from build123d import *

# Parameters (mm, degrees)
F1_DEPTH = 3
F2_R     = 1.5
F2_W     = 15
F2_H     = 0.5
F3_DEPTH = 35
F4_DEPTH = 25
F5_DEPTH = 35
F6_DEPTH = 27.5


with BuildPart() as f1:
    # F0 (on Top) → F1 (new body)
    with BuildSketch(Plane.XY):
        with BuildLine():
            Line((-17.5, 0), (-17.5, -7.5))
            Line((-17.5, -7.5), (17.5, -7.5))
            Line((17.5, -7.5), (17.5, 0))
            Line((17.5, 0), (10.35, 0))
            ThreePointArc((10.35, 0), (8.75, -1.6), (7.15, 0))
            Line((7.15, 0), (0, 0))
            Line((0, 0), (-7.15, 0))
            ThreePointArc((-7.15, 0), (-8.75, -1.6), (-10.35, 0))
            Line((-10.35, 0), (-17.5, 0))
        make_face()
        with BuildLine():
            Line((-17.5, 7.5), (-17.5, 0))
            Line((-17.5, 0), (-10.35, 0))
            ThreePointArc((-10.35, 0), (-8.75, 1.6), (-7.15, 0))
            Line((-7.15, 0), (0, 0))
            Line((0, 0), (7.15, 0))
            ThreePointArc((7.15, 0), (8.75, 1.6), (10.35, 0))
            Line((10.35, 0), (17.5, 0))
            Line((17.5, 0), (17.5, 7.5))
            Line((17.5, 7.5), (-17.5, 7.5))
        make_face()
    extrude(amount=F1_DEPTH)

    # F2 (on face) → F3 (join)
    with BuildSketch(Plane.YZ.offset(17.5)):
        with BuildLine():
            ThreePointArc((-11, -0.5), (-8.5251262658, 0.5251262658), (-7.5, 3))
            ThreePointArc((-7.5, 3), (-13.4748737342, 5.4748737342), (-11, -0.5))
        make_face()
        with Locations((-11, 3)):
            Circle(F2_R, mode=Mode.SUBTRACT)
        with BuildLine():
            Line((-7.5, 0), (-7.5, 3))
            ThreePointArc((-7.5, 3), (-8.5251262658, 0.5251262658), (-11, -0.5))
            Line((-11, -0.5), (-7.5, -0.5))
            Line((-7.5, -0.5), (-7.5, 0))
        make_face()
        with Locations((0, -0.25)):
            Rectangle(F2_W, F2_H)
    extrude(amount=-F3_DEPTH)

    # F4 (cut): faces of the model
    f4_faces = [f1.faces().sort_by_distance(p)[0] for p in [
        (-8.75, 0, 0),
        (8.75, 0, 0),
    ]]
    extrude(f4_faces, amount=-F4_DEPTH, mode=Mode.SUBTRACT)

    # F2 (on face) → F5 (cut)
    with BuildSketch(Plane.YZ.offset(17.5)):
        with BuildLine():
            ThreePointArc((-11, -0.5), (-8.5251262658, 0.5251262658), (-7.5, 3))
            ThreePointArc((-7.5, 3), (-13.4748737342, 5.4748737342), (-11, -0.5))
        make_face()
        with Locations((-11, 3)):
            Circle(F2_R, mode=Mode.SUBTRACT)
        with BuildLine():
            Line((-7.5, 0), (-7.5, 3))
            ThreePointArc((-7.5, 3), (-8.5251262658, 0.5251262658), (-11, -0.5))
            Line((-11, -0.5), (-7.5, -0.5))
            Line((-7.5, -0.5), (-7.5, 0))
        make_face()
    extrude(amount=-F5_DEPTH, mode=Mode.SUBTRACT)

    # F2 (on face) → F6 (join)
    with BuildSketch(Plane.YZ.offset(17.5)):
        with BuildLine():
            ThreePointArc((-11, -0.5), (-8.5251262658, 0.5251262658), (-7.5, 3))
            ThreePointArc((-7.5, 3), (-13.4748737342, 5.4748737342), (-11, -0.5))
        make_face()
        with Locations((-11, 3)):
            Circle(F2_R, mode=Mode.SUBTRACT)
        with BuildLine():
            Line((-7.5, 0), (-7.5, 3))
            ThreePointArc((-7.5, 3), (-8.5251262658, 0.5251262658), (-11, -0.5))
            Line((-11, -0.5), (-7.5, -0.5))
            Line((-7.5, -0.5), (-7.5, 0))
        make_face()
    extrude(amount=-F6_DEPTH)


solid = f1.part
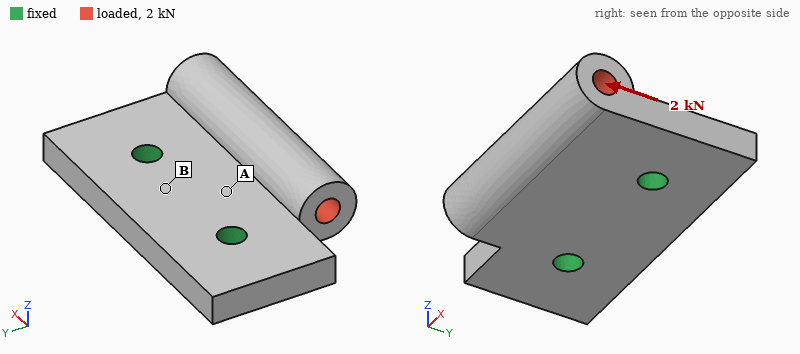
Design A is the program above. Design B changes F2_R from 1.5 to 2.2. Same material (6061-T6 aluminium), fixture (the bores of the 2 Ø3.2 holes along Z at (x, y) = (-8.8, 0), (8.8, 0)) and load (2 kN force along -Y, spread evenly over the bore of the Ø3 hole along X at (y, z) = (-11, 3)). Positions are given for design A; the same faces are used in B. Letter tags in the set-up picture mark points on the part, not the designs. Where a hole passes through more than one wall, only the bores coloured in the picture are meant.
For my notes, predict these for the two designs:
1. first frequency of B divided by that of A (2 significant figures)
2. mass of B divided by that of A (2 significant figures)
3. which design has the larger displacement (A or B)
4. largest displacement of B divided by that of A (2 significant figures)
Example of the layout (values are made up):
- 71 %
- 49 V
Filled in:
- 1.1
- 0.92
- B
- 1.2
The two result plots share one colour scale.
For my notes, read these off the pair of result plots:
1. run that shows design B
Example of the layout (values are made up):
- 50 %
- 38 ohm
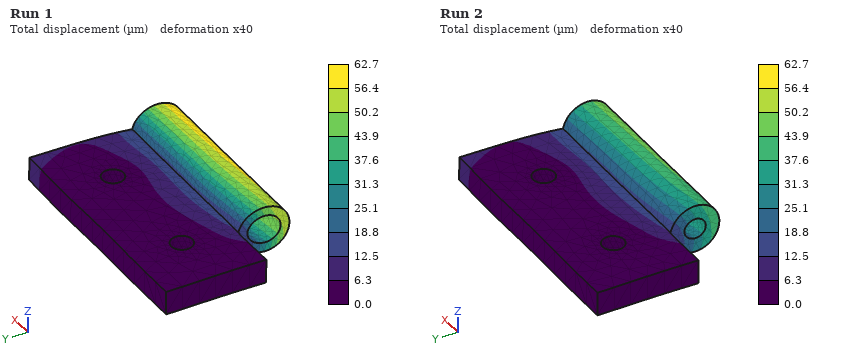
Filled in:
- Run 1
